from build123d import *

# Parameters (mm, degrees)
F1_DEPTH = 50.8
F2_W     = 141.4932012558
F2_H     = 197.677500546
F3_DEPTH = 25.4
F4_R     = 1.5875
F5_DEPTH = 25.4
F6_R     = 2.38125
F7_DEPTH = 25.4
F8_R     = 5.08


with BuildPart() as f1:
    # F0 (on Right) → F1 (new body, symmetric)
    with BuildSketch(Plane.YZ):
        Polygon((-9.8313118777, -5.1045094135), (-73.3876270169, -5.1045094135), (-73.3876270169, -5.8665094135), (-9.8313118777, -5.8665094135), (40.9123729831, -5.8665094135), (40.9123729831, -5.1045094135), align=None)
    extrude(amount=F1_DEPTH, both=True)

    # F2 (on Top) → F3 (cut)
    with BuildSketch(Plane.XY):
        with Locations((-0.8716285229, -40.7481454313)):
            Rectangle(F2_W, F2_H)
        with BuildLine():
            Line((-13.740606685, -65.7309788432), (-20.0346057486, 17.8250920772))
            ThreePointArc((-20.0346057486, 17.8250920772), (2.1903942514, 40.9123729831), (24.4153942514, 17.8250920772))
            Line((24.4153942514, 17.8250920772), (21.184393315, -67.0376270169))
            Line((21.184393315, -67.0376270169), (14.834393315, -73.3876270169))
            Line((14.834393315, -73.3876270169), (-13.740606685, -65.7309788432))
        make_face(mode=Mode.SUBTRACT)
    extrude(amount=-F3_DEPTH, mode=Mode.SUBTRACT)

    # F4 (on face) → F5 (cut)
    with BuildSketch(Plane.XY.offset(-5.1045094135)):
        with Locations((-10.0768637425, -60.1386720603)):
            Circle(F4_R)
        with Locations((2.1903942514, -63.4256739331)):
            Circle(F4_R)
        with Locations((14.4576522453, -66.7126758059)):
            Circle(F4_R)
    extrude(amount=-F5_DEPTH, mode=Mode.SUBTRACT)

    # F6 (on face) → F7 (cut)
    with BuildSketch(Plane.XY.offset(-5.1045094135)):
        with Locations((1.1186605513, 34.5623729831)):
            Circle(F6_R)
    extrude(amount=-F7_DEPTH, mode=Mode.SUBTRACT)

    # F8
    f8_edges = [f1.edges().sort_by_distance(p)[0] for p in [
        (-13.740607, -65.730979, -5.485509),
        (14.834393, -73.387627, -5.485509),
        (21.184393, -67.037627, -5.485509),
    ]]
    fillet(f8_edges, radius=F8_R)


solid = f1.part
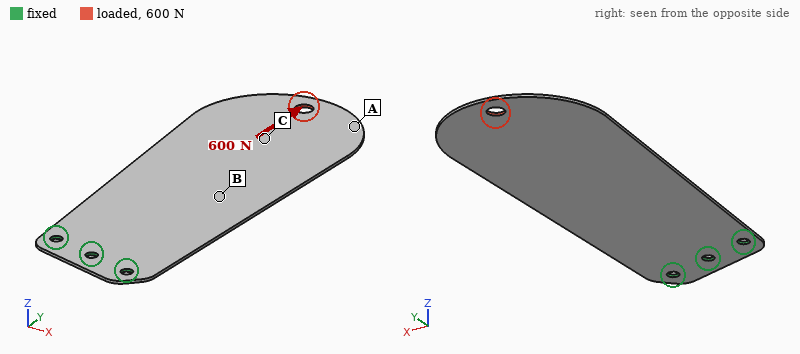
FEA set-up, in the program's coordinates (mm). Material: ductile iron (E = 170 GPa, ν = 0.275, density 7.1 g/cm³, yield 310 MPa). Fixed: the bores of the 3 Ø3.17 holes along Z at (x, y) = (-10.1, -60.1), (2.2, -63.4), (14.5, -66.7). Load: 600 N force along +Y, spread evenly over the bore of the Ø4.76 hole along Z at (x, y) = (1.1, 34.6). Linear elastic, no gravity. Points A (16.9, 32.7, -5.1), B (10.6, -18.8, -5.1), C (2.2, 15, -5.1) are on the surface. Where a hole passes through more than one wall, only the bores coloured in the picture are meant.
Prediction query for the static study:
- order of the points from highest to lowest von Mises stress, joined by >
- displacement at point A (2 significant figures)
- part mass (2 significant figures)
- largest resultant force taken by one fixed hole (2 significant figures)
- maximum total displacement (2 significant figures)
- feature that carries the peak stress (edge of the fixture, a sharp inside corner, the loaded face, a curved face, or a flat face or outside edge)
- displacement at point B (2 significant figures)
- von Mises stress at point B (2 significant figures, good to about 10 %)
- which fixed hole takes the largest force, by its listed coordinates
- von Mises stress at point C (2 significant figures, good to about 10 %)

C > B > A
10 µm
23 g
230 N
17 µm
the loaded face
5.2 µm
18 MPa
(-10.1, -60.1)
28 MPa
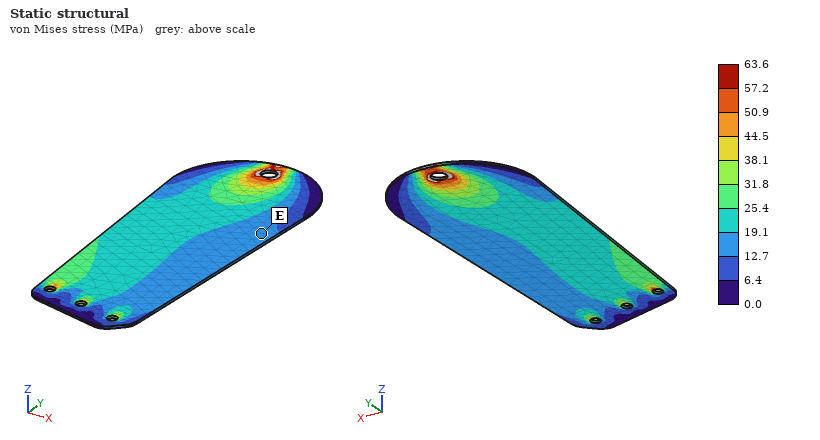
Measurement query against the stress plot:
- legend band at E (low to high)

12.7 to 19.1 MPa
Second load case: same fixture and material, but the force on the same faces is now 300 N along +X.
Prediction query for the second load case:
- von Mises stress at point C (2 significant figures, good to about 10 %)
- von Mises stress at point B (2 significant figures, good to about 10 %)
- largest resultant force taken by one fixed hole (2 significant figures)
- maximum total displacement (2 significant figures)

23 MPa
39 MPa
1.2 kN
0.20 mm
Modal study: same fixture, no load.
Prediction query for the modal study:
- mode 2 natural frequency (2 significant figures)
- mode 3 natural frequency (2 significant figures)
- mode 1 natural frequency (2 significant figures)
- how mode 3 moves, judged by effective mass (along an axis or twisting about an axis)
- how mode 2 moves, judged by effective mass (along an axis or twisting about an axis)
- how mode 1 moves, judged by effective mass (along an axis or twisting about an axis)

300 Hz
380 Hz
59 Hz
along Z
twisting about Y
along Z
